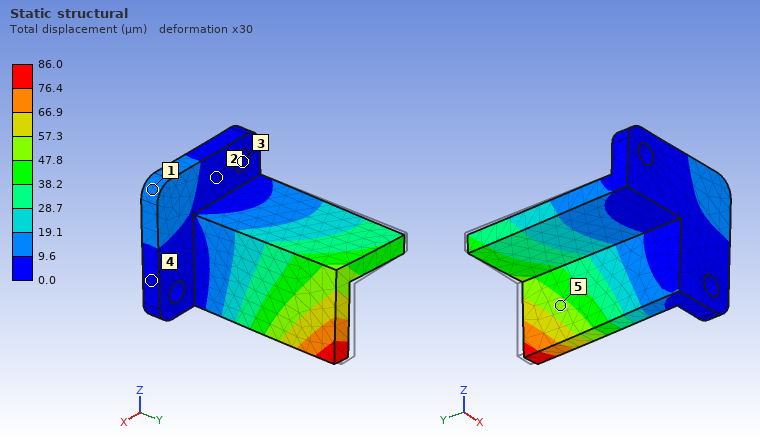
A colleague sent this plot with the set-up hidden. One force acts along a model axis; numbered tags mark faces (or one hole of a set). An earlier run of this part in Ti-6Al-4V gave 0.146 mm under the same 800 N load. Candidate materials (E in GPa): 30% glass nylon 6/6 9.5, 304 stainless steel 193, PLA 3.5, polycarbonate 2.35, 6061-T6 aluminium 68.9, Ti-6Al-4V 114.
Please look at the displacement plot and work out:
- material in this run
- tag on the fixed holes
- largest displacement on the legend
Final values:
304 stainless steel
3
86.0 µm
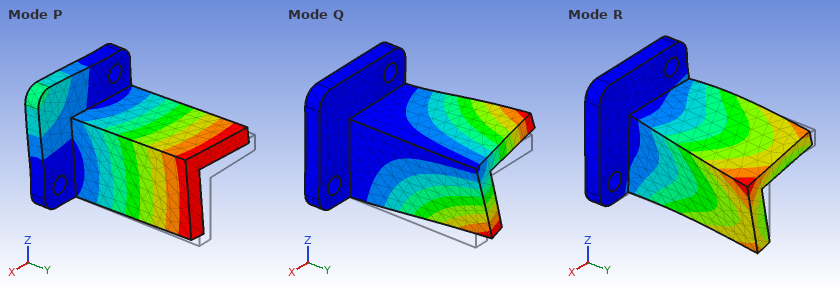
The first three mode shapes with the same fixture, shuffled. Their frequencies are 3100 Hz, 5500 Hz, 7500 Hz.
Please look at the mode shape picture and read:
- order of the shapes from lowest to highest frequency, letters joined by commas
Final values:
P, Q, R
